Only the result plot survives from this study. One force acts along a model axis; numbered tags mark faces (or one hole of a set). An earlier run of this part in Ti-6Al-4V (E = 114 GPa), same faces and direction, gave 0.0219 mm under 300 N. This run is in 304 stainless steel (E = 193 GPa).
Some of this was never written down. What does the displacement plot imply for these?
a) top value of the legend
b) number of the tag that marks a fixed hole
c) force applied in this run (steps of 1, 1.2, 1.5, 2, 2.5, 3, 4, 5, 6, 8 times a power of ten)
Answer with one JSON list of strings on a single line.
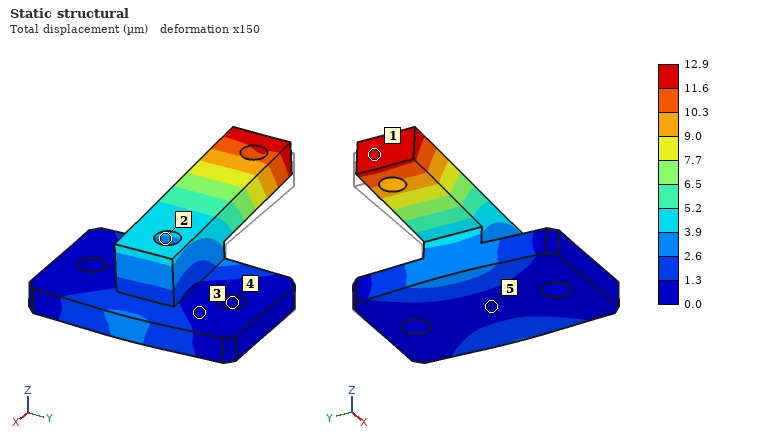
["12.9 µm", "4", "300 N"]
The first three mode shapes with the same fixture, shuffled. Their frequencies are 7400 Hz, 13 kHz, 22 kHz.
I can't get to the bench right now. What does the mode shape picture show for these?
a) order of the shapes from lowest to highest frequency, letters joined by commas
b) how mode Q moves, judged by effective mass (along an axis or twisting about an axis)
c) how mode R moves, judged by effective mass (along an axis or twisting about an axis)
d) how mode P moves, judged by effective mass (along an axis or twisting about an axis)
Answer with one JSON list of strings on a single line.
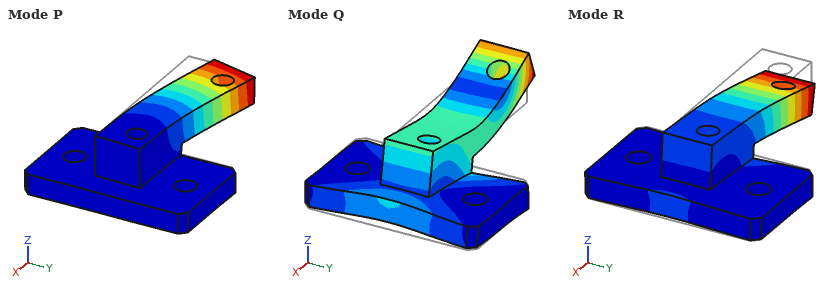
["R, P, Q", "along X", "along Z", "along Y"]
